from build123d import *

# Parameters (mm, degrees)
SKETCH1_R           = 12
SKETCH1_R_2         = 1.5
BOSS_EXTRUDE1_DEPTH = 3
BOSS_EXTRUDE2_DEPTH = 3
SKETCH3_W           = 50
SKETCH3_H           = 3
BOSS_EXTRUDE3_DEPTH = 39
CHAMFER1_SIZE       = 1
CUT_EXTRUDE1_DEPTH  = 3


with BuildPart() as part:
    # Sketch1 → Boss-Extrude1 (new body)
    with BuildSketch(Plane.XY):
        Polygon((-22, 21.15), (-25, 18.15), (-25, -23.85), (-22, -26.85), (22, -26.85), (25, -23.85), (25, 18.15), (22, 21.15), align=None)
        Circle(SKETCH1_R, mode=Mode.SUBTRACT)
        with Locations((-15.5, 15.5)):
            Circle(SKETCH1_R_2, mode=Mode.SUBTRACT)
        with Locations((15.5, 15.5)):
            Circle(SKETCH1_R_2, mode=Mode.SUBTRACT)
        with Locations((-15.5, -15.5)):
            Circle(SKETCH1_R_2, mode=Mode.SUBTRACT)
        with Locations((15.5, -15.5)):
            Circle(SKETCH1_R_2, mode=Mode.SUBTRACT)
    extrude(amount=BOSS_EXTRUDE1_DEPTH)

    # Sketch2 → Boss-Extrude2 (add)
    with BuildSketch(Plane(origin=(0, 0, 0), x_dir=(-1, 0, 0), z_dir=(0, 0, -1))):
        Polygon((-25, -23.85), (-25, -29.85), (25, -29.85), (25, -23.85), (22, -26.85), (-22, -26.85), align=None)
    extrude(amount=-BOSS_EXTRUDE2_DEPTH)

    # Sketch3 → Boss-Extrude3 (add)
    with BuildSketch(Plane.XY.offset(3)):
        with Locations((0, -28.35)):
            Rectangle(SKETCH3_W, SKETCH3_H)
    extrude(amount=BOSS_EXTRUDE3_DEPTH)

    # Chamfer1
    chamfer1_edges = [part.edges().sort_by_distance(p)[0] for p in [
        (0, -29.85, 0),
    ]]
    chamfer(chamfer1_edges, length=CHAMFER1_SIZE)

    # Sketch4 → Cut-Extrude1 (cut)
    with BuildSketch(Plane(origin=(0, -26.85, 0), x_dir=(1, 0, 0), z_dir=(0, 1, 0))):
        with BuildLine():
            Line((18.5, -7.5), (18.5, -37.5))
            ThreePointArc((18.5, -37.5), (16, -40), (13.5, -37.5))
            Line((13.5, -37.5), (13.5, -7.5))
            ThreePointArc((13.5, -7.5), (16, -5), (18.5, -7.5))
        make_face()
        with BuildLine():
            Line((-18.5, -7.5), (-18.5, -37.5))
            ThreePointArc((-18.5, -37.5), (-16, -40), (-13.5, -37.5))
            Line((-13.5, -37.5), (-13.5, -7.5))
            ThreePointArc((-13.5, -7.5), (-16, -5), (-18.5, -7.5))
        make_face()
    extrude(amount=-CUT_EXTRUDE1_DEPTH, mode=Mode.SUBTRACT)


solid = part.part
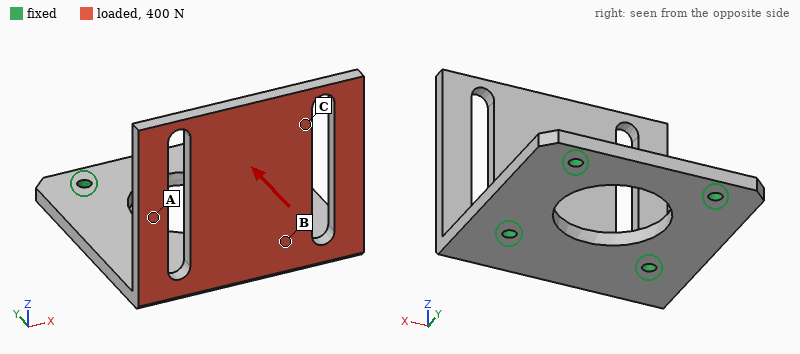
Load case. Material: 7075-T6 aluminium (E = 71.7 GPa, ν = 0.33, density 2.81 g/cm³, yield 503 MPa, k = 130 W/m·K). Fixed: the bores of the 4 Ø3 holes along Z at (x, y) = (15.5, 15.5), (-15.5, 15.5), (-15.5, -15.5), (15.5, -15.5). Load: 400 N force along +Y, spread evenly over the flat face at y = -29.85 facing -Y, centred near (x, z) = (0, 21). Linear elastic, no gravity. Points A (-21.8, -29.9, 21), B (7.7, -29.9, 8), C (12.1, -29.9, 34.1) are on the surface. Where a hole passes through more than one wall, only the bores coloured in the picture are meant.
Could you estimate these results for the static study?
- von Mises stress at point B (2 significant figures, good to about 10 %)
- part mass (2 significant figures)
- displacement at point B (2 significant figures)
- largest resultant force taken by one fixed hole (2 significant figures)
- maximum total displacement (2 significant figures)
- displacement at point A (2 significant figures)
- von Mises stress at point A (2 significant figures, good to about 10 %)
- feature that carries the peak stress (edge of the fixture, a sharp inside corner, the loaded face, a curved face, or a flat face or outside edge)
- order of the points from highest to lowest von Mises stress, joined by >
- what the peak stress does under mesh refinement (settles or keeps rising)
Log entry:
85 MPa
31 g
0.16 mm
200 N
0.97 mm
0.41 mm
37 MPa
edge of the fixture
B > A > C
keeps rising
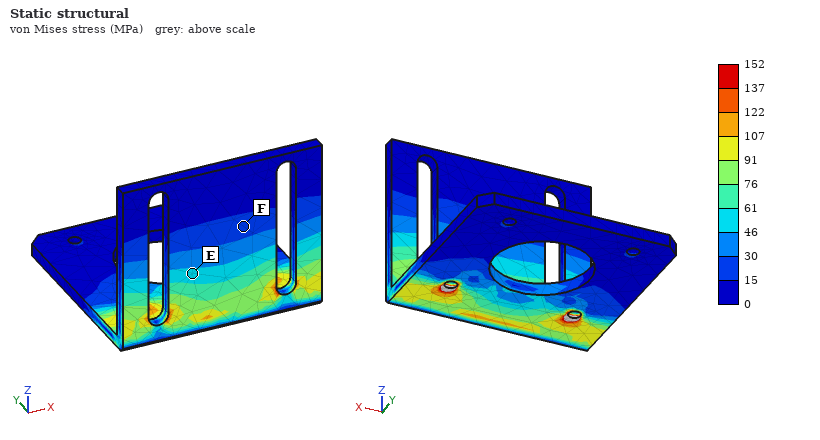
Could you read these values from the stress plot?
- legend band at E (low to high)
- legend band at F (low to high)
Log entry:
46 to 61 MPa
15 to 30 MPa
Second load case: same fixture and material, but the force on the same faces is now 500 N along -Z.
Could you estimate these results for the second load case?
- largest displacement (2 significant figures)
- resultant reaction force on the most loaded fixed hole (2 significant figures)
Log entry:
0.36 mm
270 N
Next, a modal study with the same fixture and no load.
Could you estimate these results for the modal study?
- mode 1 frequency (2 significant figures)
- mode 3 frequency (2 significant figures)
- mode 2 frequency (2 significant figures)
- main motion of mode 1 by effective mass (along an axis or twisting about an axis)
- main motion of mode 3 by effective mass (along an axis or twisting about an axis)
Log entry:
1000 Hz
3400 Hz
2400 Hz
along Y
along X
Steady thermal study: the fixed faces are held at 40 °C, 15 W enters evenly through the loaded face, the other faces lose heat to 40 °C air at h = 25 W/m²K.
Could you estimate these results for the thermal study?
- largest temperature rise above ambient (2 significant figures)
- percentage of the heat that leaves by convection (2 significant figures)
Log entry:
28 K
11 %
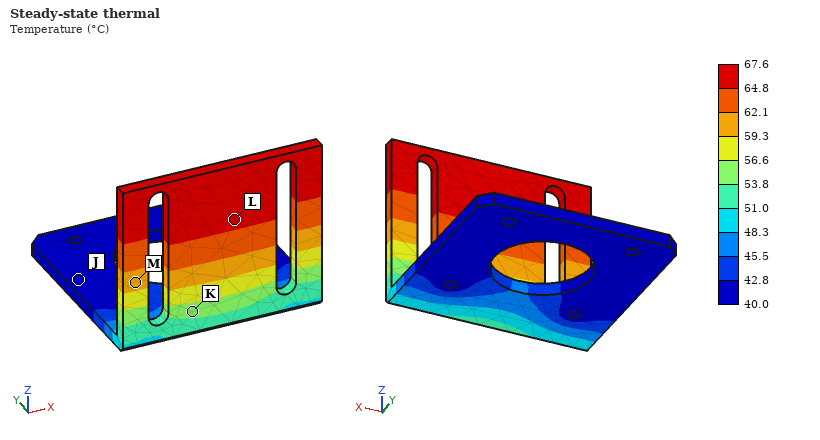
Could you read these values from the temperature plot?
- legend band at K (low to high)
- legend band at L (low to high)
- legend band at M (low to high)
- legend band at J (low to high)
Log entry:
53.8 to 56.6 °C
64.8 to 67.6 °C
59.3 to 62.1 °C
40.0 to 42.8 °C
